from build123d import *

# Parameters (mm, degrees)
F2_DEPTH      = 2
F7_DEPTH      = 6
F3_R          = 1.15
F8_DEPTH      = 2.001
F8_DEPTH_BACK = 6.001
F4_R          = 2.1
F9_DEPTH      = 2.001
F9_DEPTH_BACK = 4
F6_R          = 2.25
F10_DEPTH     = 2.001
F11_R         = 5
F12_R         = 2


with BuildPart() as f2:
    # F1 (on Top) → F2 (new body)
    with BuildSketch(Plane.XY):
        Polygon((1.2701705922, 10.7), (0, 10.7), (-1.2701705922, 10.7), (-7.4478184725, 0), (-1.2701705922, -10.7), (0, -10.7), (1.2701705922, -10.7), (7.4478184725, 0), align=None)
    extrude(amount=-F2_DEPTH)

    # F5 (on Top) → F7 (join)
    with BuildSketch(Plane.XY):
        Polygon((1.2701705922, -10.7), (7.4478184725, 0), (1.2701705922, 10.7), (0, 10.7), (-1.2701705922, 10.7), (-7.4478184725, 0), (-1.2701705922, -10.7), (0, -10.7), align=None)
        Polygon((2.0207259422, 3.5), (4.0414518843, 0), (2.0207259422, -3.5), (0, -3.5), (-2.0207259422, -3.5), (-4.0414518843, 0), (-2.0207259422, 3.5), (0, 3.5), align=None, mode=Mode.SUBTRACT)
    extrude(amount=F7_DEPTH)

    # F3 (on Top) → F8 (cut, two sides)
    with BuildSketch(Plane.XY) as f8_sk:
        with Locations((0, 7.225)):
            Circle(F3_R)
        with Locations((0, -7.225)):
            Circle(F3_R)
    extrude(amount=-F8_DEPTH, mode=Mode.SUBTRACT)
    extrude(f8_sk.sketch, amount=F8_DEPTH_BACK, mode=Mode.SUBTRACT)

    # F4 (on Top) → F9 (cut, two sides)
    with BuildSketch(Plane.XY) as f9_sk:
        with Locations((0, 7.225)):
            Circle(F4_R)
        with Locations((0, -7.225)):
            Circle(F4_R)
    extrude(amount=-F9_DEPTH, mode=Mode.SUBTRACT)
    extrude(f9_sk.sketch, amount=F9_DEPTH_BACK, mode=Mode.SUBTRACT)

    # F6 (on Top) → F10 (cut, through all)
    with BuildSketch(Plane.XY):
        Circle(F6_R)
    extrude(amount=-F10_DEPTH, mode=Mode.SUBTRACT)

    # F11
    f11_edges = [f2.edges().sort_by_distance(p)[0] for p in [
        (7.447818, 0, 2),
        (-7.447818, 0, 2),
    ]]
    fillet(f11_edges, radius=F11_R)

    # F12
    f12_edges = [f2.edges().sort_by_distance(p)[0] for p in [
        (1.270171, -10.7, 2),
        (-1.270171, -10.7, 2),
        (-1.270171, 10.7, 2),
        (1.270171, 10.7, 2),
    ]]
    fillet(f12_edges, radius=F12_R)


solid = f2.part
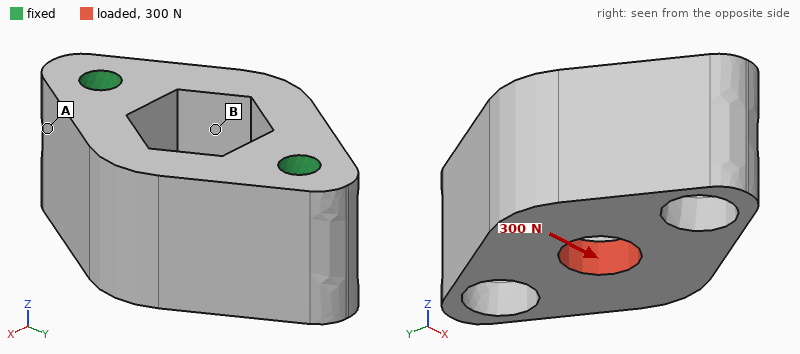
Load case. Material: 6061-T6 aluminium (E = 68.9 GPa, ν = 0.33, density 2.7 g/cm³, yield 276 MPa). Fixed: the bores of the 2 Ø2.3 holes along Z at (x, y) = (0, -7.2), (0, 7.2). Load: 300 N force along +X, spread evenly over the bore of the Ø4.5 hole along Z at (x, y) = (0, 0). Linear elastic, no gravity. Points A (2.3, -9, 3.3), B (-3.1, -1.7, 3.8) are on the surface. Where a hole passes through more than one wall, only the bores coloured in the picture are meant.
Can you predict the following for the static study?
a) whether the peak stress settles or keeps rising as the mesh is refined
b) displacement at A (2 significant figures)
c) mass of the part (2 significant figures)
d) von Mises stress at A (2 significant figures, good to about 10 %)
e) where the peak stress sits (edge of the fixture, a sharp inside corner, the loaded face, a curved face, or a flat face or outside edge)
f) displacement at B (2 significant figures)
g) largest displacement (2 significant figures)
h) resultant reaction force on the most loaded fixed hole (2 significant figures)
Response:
keeps rising
3.6 µm
2.7 g
24 MPa
edge of the fixture
5.8 µm
19 µm
150 N
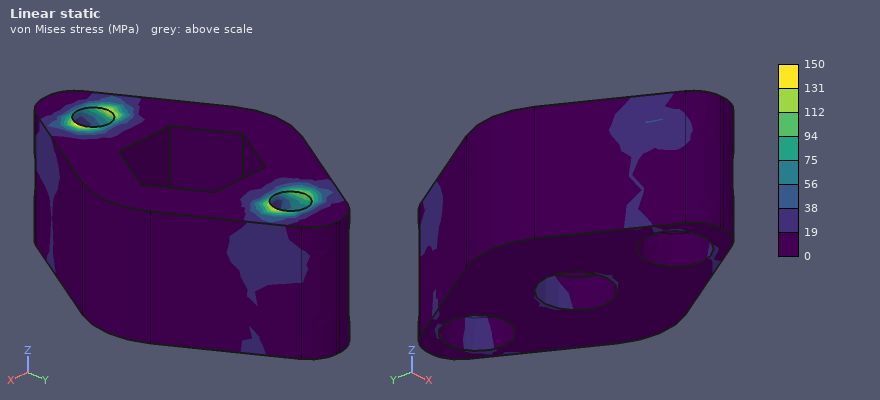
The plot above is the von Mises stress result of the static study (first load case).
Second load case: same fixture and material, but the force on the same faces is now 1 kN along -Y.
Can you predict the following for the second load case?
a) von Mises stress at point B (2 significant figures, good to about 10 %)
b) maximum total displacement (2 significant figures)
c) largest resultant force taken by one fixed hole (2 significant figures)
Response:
25 MPa
9.5 µm
630 N
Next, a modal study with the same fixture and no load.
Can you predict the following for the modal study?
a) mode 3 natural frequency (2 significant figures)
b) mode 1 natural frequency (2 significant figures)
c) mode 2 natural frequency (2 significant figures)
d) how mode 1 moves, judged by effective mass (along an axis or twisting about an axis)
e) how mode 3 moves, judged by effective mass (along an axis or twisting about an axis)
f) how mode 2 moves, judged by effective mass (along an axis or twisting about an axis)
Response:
53 kHz
19 kHz
49 kHz
along X
along Y
along Z
